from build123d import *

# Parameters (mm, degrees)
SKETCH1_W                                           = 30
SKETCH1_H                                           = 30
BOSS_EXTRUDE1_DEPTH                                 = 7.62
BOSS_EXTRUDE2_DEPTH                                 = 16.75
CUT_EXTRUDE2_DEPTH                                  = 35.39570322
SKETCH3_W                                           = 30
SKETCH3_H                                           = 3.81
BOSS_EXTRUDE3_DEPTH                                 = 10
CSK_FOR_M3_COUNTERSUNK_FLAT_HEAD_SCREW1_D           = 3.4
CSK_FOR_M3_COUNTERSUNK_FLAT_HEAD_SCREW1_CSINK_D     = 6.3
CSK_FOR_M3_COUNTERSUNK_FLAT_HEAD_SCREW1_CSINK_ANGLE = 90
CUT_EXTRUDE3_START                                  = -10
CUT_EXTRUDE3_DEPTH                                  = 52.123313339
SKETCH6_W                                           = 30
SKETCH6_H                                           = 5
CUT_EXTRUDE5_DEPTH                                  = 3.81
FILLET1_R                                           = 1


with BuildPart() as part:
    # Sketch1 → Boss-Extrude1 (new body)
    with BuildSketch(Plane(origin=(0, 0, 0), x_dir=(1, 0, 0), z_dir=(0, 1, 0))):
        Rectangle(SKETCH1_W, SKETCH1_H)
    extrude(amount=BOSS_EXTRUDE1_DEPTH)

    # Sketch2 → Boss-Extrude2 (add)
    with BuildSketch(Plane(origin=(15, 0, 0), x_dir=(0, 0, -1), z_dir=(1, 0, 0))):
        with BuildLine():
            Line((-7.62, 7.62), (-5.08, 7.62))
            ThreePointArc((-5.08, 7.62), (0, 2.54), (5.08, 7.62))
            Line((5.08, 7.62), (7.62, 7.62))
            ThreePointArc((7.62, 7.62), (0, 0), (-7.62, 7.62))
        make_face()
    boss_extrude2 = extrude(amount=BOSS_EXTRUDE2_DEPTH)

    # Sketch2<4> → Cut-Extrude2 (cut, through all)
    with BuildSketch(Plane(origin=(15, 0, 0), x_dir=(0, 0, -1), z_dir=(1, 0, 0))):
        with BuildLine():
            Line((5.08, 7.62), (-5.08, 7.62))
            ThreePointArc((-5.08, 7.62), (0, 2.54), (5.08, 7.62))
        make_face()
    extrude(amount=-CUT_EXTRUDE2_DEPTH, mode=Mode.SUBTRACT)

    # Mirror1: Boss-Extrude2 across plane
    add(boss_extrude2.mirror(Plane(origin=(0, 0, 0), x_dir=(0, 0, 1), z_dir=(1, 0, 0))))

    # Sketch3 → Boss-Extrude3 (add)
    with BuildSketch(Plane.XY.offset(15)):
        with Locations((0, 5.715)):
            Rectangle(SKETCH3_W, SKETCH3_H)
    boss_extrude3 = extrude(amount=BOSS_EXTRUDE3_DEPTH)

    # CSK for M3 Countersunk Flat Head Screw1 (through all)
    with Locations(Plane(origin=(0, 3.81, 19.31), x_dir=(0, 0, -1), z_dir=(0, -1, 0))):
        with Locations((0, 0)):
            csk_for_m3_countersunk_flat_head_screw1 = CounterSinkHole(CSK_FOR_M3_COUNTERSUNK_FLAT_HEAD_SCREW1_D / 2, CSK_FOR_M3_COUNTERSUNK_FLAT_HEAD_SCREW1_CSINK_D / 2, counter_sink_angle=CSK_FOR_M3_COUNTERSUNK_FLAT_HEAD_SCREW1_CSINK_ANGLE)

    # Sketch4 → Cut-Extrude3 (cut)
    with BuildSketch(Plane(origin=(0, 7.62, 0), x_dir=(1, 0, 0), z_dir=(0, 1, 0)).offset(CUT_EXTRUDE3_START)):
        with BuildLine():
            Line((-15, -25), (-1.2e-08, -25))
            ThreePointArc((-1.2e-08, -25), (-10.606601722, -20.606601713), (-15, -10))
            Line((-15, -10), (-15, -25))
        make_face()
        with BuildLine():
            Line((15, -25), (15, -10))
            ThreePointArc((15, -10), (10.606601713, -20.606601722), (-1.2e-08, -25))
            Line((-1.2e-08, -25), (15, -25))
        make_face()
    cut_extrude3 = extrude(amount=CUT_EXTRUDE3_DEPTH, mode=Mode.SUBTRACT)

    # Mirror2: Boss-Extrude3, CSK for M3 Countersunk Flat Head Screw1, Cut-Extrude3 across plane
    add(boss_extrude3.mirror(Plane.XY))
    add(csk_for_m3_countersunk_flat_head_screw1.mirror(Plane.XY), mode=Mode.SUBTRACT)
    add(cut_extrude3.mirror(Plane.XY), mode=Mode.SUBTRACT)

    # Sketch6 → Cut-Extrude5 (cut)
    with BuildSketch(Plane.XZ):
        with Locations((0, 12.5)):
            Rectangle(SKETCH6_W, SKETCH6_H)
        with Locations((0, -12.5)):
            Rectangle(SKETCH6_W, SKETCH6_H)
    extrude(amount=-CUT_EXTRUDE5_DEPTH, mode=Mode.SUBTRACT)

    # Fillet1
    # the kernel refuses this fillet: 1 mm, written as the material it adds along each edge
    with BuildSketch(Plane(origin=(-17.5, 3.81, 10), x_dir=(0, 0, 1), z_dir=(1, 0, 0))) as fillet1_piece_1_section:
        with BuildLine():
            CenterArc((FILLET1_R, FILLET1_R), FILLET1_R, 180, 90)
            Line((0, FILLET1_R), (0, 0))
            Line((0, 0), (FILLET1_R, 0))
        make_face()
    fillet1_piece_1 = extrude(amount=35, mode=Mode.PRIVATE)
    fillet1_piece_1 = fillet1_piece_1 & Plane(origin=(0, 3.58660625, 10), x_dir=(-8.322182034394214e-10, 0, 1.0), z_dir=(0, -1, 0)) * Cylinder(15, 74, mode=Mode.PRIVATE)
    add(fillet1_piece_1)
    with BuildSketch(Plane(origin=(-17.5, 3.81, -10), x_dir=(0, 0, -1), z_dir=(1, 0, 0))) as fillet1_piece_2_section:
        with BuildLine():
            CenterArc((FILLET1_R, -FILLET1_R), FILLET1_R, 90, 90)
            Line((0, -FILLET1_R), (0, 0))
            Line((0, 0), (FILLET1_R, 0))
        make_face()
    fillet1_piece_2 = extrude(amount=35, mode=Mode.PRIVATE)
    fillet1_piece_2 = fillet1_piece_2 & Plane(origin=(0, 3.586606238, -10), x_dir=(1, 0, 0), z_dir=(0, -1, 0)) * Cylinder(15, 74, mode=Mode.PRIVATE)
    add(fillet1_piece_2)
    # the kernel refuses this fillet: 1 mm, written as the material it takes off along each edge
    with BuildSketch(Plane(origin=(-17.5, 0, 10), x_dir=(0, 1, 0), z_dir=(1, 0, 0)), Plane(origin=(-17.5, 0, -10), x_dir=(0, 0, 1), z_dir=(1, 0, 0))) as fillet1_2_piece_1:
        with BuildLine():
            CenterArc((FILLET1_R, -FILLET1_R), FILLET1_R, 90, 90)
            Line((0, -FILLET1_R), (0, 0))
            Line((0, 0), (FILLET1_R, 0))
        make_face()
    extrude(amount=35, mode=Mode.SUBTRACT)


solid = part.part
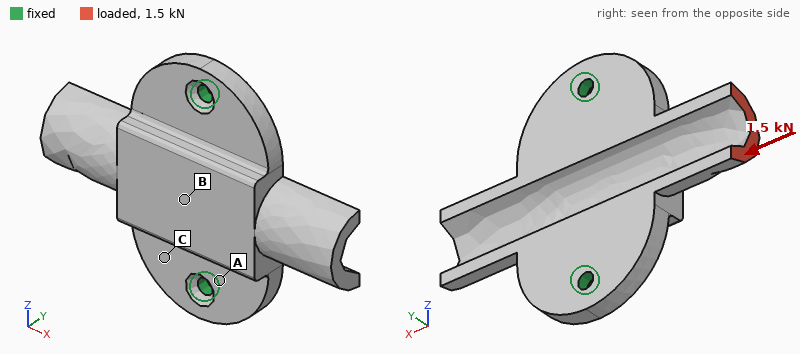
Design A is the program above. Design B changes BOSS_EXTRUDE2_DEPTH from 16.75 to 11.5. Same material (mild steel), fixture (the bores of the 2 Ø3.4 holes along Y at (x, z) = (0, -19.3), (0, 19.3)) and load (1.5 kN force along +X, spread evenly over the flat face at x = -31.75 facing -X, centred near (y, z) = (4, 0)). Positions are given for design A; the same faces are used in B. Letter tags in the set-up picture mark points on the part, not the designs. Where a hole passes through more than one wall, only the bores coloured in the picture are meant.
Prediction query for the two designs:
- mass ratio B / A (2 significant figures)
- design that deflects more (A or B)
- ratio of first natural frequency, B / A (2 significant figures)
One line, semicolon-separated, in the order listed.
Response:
0.93; A; 1.2
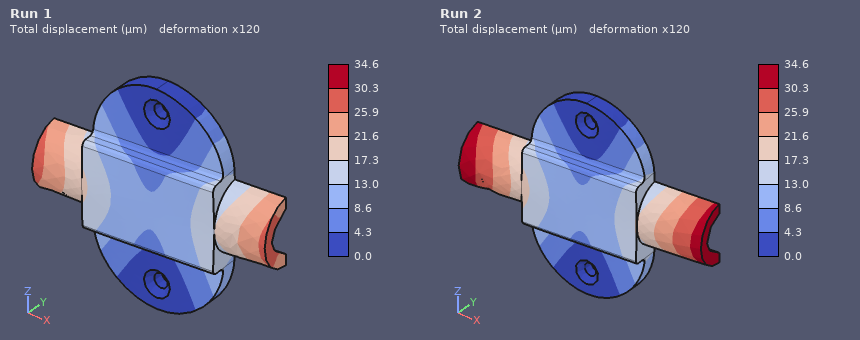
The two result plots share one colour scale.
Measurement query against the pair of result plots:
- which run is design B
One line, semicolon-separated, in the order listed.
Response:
Run 1
